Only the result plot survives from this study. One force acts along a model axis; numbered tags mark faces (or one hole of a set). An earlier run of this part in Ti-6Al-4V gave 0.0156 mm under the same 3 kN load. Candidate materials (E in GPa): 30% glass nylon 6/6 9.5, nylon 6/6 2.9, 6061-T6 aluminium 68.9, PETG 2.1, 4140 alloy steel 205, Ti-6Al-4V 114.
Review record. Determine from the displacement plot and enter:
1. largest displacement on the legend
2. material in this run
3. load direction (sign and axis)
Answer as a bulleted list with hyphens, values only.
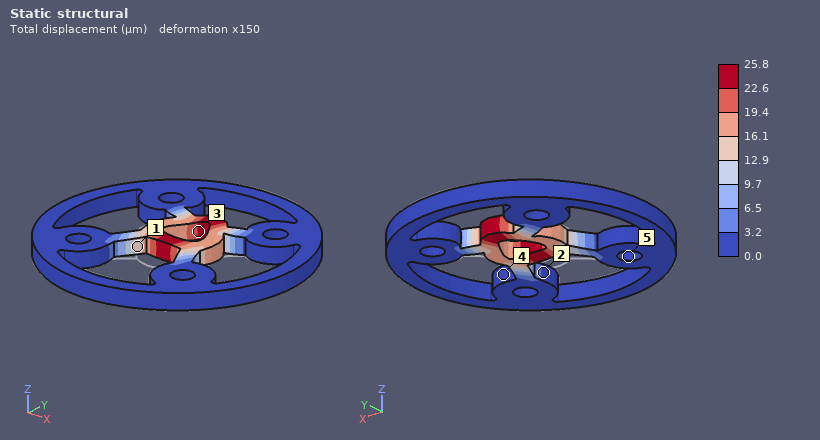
- 25.8 µm
- 6061-T6 aluminium
- +Y
